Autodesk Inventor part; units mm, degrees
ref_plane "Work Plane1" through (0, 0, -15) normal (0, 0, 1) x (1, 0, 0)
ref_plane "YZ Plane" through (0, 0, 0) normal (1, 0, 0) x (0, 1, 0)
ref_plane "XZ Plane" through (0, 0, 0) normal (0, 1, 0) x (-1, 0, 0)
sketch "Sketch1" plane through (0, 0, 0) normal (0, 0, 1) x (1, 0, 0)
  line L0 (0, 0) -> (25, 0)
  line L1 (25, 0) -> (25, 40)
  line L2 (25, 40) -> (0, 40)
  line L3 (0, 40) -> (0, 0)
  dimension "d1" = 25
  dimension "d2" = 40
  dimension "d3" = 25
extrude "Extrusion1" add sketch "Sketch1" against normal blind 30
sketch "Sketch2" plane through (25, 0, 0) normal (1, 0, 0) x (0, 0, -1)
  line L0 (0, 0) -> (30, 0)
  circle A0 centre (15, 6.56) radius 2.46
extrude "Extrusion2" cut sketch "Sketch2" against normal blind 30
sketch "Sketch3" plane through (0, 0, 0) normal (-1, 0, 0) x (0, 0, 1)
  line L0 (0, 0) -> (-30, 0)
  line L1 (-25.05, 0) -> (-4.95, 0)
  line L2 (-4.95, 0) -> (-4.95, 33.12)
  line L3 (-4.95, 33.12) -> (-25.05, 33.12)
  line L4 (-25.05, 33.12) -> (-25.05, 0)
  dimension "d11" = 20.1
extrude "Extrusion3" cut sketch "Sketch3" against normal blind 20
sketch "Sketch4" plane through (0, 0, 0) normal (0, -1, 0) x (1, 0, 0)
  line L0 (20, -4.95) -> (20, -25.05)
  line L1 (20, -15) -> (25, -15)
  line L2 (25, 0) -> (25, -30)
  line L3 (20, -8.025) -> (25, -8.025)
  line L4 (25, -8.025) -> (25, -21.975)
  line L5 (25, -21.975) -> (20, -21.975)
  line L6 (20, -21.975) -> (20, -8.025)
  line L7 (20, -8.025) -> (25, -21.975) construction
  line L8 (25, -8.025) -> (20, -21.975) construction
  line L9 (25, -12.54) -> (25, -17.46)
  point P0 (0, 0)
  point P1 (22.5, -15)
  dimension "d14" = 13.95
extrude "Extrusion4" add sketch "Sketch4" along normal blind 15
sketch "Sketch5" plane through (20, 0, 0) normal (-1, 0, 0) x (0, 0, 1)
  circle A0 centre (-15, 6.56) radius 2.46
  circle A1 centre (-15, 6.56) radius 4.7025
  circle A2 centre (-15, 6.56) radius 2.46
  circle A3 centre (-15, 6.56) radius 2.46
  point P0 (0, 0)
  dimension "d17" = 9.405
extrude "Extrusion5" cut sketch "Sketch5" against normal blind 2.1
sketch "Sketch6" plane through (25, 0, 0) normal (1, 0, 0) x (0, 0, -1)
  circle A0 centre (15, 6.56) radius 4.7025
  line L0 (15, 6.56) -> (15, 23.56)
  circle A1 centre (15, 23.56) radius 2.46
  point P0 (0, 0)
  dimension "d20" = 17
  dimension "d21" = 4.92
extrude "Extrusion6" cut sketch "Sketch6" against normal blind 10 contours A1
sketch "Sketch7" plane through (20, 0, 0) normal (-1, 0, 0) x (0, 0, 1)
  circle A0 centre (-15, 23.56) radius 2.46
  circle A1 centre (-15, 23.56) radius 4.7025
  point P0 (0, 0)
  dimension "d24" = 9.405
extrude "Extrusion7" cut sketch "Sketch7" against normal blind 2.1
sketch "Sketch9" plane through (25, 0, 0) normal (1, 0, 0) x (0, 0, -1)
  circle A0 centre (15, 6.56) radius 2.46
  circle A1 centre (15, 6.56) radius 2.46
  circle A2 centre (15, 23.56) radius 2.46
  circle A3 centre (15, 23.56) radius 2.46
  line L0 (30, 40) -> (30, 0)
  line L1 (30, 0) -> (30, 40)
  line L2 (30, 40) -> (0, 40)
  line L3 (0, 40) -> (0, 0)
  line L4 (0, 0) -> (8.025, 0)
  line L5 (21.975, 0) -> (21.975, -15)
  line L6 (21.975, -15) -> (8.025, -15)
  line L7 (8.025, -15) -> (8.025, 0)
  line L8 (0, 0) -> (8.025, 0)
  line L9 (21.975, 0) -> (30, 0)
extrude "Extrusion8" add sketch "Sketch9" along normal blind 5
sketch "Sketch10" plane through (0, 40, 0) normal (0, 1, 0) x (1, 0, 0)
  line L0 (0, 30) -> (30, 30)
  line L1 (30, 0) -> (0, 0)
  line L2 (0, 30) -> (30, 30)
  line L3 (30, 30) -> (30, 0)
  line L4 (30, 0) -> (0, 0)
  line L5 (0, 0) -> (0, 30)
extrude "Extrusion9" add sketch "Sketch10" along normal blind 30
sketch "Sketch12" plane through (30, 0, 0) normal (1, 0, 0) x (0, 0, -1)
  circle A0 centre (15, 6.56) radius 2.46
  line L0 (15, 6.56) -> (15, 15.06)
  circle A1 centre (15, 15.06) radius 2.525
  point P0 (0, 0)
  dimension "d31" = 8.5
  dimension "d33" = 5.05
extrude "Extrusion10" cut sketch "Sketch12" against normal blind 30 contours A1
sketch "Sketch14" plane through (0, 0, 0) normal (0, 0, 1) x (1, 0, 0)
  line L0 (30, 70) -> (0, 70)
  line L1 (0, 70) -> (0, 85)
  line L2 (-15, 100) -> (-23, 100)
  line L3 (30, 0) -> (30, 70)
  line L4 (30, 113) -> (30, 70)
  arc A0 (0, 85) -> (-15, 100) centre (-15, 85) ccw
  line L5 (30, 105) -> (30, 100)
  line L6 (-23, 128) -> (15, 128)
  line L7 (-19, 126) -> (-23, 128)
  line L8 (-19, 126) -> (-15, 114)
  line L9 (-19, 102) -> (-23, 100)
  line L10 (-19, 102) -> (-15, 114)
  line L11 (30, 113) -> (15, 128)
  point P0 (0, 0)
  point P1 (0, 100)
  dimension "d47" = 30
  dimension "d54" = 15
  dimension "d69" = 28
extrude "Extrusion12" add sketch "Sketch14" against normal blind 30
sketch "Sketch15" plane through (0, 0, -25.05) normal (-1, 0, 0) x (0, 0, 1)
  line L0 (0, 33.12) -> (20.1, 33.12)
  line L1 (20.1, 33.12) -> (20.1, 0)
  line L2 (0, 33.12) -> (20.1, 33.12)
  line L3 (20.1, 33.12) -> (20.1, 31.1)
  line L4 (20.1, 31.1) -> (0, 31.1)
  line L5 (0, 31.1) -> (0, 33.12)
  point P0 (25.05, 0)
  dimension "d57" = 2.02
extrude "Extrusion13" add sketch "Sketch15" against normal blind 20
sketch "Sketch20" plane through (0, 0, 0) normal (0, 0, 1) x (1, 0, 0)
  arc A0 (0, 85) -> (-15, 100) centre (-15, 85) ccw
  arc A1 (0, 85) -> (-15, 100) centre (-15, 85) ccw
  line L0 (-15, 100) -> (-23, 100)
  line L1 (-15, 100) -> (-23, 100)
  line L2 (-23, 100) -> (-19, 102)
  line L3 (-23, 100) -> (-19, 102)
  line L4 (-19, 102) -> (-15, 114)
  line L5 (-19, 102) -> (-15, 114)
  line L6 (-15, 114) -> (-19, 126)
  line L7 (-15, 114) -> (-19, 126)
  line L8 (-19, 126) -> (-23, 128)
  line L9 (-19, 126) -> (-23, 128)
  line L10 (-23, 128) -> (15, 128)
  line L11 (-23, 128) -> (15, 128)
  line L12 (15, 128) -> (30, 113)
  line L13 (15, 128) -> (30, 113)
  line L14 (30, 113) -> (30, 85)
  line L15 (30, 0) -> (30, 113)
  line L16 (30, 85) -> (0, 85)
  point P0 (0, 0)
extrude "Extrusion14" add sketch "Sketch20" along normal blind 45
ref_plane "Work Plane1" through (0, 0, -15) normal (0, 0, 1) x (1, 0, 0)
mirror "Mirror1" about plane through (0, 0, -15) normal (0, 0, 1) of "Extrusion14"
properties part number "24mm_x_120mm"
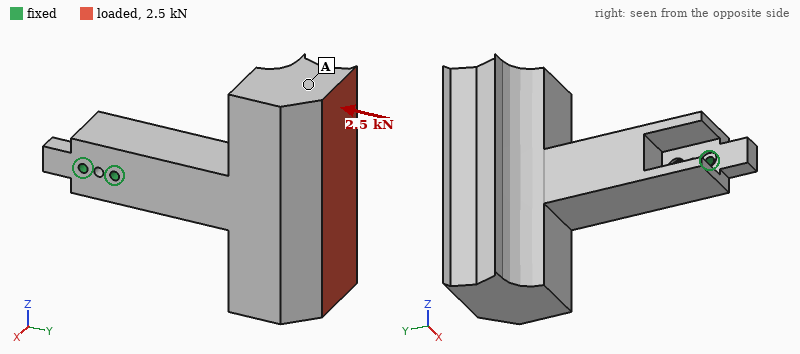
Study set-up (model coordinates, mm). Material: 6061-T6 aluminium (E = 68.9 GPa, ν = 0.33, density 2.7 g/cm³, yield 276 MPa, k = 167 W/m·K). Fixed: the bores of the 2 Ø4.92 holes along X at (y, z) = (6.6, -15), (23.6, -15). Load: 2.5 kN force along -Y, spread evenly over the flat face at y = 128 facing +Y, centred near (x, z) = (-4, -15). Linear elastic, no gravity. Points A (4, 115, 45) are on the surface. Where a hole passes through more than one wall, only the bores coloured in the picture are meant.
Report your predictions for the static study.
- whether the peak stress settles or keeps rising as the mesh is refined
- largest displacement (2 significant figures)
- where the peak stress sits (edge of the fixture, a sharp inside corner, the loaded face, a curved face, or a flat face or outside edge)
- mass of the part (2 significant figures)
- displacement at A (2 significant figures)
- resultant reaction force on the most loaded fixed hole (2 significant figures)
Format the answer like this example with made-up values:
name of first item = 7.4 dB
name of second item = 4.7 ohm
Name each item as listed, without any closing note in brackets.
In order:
whether the peak stress settles or keeps rising as the mesh is refined = keeps rising
largest displacement = 0.24 mm
where the peak stress sits = edge of the fixture
mass of the part = 730 g
displacement at A = 0.19 mm
resultant reaction force on the most loaded fixed hole = 3.4 kN
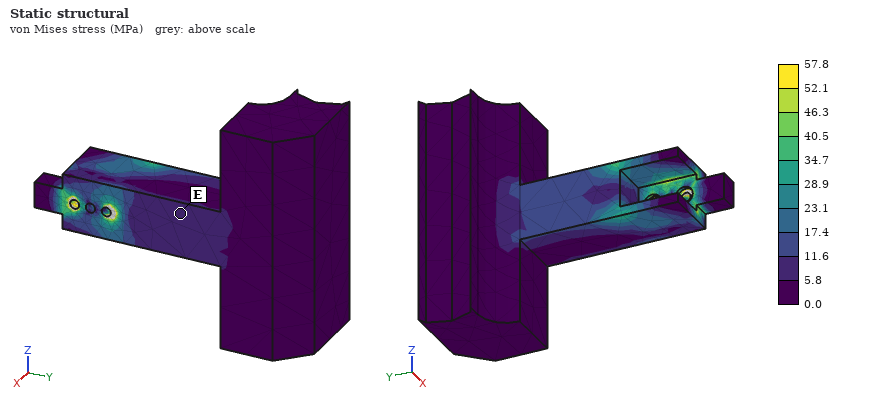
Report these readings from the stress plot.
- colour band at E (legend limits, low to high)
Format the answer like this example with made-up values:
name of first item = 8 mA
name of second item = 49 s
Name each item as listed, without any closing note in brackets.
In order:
colour band at E = 5.8 to 11.6 MPa
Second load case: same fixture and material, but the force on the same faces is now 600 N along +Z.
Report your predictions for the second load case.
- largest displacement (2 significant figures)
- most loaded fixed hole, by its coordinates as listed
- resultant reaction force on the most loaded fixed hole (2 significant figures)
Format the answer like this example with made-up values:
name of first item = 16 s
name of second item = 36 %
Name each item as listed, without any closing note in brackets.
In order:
largest displacement = 0.19 mm
most loaded fixed hole, by its coordinates as listed = (23.6, -15)
resultant reaction force on the most loaded fixed hole = 3.3 kN
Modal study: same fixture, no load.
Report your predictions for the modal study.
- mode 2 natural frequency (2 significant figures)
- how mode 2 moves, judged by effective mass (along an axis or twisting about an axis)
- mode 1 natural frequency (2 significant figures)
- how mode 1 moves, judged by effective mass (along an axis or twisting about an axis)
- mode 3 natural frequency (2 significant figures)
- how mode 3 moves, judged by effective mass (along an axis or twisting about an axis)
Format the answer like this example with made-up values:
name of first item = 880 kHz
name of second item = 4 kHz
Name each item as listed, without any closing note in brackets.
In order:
mode 2 natural frequency = 490 Hz
how mode 2 moves, judged by effective mass = along Z
mode 1 natural frequency = 460 Hz
how mode 1 moves, judged by effective mass = along X
mode 3 natural frequency = 700 Hz
how mode 3 moves, judged by effective mass = twisting about Y
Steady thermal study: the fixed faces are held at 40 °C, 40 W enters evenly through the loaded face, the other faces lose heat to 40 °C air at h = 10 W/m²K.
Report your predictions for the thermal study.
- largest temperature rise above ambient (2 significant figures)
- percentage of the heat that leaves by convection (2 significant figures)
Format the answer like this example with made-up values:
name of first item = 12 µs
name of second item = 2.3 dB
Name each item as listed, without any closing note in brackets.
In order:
largest temperature rise above ambient = 26 K
percentage of the heat that leaves by convection = 15 %
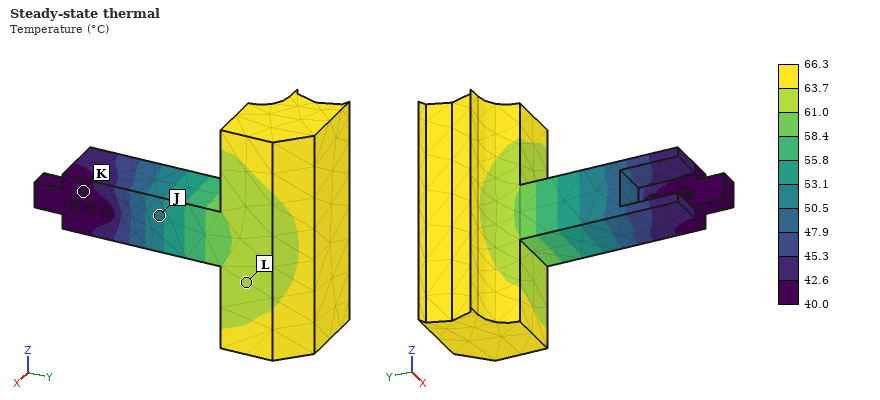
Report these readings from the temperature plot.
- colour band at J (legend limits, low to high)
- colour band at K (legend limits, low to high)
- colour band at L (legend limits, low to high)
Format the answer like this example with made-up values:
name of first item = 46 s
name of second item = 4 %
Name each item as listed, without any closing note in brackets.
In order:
colour band at J = 50.5 to 53.1 °C
colour band at K = 40.0 to 42.6 °C
colour band at L = 61.0 to 63.7 °C
